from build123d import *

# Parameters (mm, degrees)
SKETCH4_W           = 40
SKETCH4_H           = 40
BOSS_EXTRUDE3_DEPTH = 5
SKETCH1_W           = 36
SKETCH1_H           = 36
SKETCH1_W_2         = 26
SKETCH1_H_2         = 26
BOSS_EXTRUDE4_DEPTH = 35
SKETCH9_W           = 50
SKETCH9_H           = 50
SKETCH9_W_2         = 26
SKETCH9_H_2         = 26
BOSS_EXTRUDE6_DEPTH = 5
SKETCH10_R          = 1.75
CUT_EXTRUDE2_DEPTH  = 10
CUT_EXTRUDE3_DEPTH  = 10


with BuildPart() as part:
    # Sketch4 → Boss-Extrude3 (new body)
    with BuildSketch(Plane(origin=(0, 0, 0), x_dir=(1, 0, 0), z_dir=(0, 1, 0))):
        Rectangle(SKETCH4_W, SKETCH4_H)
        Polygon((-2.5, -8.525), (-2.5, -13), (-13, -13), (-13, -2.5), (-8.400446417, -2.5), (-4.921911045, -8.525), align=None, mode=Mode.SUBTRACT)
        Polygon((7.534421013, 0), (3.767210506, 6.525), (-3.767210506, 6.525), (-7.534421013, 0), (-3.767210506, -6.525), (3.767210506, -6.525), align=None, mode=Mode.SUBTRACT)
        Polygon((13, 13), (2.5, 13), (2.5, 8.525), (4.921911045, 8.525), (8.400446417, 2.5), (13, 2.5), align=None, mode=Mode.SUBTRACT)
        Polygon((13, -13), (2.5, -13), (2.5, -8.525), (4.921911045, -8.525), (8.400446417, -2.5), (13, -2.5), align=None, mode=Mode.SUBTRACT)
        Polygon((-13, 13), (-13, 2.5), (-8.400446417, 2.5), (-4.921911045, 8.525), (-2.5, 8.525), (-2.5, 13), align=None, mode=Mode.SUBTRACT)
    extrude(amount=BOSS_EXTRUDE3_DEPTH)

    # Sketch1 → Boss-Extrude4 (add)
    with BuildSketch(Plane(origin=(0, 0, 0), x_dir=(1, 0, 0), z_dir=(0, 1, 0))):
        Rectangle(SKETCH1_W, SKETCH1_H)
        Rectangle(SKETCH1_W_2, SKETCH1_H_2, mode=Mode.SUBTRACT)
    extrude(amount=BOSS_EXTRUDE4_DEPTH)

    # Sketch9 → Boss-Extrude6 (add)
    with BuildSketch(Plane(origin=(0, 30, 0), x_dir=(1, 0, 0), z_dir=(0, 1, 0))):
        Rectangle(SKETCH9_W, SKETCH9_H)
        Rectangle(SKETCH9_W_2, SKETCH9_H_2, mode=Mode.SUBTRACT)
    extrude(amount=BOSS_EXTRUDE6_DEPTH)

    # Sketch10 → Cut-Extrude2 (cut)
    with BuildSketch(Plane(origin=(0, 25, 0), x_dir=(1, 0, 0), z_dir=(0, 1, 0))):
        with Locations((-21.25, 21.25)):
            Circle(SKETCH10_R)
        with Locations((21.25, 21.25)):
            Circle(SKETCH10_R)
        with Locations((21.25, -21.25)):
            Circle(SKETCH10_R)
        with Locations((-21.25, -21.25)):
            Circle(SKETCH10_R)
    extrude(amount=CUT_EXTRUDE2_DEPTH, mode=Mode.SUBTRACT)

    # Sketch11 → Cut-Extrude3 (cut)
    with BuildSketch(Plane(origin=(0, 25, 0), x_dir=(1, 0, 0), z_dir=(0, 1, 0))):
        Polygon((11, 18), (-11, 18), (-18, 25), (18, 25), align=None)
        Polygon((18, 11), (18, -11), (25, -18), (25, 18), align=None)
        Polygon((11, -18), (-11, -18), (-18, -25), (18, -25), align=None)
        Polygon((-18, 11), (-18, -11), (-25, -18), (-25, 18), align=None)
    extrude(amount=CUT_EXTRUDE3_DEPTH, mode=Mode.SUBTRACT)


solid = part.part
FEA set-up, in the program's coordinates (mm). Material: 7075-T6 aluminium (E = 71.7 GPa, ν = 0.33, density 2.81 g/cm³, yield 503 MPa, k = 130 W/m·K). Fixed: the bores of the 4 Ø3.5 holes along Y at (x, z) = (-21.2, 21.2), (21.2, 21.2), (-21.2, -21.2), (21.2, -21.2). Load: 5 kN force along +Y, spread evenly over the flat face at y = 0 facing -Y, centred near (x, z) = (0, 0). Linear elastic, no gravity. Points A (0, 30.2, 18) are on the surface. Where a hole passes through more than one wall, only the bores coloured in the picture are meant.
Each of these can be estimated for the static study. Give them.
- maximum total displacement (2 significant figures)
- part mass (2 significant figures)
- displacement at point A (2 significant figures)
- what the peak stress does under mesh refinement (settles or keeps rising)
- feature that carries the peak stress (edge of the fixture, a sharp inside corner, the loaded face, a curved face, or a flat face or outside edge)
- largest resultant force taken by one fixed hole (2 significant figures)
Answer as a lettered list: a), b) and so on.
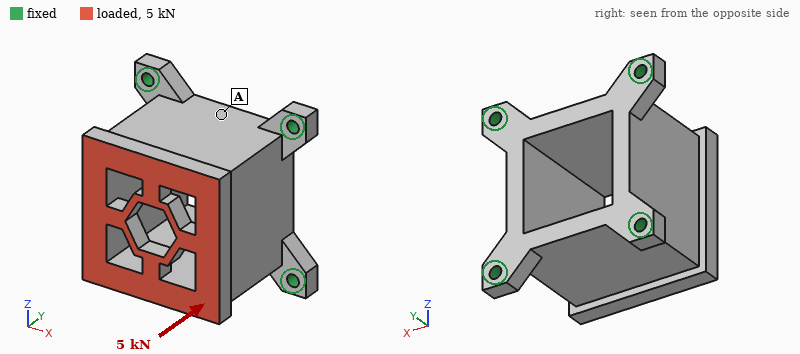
a) 28 µm
b) 73 g
c) 20 µm
d) keeps rising
e) edge of the fixture
f) 1.4 kN
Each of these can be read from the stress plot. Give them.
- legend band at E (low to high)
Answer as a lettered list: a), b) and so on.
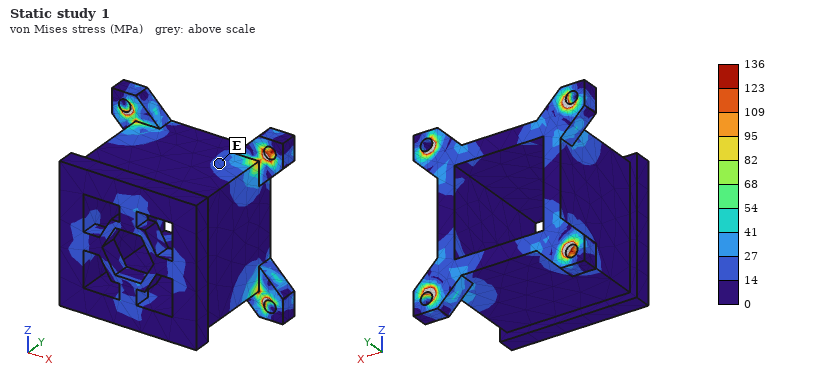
a) 14 to 27 MPa
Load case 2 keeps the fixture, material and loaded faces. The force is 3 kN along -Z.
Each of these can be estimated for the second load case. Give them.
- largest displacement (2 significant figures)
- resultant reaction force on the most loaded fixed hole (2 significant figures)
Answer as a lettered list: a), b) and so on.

a) 58 µm
b) 1.6 kN
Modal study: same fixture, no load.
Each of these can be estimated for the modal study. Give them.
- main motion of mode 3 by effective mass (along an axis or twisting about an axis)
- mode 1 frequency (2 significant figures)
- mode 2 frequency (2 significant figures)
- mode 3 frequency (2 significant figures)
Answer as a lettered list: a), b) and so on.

a) along Y
b) 7200 Hz
c) 7200 Hz
d) 9800 Hz
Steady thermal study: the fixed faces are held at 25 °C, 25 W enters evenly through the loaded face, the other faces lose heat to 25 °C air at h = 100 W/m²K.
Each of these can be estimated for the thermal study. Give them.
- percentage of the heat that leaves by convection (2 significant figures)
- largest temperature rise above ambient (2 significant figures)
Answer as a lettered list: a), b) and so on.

a) 38 %
b) 14 K
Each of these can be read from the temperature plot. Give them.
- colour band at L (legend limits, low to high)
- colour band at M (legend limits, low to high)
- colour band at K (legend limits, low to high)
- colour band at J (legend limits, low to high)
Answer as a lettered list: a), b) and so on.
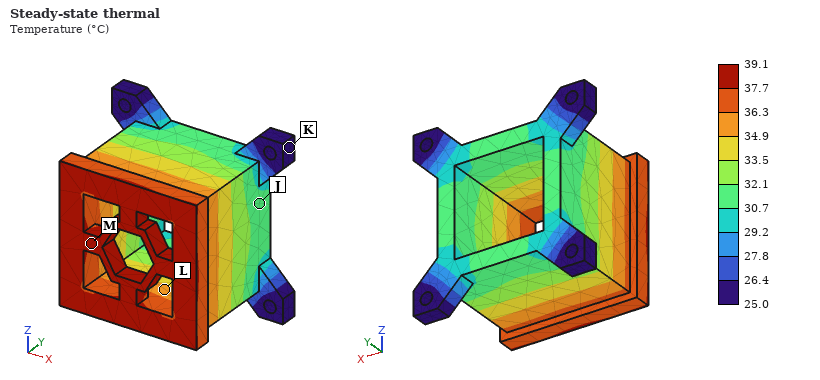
a) 34.9 to 36.3 °C
b) 37.7 to 39.1 °C
c) 25.0 to 26.4 °C
d) 30.7 to 32.1 °C
